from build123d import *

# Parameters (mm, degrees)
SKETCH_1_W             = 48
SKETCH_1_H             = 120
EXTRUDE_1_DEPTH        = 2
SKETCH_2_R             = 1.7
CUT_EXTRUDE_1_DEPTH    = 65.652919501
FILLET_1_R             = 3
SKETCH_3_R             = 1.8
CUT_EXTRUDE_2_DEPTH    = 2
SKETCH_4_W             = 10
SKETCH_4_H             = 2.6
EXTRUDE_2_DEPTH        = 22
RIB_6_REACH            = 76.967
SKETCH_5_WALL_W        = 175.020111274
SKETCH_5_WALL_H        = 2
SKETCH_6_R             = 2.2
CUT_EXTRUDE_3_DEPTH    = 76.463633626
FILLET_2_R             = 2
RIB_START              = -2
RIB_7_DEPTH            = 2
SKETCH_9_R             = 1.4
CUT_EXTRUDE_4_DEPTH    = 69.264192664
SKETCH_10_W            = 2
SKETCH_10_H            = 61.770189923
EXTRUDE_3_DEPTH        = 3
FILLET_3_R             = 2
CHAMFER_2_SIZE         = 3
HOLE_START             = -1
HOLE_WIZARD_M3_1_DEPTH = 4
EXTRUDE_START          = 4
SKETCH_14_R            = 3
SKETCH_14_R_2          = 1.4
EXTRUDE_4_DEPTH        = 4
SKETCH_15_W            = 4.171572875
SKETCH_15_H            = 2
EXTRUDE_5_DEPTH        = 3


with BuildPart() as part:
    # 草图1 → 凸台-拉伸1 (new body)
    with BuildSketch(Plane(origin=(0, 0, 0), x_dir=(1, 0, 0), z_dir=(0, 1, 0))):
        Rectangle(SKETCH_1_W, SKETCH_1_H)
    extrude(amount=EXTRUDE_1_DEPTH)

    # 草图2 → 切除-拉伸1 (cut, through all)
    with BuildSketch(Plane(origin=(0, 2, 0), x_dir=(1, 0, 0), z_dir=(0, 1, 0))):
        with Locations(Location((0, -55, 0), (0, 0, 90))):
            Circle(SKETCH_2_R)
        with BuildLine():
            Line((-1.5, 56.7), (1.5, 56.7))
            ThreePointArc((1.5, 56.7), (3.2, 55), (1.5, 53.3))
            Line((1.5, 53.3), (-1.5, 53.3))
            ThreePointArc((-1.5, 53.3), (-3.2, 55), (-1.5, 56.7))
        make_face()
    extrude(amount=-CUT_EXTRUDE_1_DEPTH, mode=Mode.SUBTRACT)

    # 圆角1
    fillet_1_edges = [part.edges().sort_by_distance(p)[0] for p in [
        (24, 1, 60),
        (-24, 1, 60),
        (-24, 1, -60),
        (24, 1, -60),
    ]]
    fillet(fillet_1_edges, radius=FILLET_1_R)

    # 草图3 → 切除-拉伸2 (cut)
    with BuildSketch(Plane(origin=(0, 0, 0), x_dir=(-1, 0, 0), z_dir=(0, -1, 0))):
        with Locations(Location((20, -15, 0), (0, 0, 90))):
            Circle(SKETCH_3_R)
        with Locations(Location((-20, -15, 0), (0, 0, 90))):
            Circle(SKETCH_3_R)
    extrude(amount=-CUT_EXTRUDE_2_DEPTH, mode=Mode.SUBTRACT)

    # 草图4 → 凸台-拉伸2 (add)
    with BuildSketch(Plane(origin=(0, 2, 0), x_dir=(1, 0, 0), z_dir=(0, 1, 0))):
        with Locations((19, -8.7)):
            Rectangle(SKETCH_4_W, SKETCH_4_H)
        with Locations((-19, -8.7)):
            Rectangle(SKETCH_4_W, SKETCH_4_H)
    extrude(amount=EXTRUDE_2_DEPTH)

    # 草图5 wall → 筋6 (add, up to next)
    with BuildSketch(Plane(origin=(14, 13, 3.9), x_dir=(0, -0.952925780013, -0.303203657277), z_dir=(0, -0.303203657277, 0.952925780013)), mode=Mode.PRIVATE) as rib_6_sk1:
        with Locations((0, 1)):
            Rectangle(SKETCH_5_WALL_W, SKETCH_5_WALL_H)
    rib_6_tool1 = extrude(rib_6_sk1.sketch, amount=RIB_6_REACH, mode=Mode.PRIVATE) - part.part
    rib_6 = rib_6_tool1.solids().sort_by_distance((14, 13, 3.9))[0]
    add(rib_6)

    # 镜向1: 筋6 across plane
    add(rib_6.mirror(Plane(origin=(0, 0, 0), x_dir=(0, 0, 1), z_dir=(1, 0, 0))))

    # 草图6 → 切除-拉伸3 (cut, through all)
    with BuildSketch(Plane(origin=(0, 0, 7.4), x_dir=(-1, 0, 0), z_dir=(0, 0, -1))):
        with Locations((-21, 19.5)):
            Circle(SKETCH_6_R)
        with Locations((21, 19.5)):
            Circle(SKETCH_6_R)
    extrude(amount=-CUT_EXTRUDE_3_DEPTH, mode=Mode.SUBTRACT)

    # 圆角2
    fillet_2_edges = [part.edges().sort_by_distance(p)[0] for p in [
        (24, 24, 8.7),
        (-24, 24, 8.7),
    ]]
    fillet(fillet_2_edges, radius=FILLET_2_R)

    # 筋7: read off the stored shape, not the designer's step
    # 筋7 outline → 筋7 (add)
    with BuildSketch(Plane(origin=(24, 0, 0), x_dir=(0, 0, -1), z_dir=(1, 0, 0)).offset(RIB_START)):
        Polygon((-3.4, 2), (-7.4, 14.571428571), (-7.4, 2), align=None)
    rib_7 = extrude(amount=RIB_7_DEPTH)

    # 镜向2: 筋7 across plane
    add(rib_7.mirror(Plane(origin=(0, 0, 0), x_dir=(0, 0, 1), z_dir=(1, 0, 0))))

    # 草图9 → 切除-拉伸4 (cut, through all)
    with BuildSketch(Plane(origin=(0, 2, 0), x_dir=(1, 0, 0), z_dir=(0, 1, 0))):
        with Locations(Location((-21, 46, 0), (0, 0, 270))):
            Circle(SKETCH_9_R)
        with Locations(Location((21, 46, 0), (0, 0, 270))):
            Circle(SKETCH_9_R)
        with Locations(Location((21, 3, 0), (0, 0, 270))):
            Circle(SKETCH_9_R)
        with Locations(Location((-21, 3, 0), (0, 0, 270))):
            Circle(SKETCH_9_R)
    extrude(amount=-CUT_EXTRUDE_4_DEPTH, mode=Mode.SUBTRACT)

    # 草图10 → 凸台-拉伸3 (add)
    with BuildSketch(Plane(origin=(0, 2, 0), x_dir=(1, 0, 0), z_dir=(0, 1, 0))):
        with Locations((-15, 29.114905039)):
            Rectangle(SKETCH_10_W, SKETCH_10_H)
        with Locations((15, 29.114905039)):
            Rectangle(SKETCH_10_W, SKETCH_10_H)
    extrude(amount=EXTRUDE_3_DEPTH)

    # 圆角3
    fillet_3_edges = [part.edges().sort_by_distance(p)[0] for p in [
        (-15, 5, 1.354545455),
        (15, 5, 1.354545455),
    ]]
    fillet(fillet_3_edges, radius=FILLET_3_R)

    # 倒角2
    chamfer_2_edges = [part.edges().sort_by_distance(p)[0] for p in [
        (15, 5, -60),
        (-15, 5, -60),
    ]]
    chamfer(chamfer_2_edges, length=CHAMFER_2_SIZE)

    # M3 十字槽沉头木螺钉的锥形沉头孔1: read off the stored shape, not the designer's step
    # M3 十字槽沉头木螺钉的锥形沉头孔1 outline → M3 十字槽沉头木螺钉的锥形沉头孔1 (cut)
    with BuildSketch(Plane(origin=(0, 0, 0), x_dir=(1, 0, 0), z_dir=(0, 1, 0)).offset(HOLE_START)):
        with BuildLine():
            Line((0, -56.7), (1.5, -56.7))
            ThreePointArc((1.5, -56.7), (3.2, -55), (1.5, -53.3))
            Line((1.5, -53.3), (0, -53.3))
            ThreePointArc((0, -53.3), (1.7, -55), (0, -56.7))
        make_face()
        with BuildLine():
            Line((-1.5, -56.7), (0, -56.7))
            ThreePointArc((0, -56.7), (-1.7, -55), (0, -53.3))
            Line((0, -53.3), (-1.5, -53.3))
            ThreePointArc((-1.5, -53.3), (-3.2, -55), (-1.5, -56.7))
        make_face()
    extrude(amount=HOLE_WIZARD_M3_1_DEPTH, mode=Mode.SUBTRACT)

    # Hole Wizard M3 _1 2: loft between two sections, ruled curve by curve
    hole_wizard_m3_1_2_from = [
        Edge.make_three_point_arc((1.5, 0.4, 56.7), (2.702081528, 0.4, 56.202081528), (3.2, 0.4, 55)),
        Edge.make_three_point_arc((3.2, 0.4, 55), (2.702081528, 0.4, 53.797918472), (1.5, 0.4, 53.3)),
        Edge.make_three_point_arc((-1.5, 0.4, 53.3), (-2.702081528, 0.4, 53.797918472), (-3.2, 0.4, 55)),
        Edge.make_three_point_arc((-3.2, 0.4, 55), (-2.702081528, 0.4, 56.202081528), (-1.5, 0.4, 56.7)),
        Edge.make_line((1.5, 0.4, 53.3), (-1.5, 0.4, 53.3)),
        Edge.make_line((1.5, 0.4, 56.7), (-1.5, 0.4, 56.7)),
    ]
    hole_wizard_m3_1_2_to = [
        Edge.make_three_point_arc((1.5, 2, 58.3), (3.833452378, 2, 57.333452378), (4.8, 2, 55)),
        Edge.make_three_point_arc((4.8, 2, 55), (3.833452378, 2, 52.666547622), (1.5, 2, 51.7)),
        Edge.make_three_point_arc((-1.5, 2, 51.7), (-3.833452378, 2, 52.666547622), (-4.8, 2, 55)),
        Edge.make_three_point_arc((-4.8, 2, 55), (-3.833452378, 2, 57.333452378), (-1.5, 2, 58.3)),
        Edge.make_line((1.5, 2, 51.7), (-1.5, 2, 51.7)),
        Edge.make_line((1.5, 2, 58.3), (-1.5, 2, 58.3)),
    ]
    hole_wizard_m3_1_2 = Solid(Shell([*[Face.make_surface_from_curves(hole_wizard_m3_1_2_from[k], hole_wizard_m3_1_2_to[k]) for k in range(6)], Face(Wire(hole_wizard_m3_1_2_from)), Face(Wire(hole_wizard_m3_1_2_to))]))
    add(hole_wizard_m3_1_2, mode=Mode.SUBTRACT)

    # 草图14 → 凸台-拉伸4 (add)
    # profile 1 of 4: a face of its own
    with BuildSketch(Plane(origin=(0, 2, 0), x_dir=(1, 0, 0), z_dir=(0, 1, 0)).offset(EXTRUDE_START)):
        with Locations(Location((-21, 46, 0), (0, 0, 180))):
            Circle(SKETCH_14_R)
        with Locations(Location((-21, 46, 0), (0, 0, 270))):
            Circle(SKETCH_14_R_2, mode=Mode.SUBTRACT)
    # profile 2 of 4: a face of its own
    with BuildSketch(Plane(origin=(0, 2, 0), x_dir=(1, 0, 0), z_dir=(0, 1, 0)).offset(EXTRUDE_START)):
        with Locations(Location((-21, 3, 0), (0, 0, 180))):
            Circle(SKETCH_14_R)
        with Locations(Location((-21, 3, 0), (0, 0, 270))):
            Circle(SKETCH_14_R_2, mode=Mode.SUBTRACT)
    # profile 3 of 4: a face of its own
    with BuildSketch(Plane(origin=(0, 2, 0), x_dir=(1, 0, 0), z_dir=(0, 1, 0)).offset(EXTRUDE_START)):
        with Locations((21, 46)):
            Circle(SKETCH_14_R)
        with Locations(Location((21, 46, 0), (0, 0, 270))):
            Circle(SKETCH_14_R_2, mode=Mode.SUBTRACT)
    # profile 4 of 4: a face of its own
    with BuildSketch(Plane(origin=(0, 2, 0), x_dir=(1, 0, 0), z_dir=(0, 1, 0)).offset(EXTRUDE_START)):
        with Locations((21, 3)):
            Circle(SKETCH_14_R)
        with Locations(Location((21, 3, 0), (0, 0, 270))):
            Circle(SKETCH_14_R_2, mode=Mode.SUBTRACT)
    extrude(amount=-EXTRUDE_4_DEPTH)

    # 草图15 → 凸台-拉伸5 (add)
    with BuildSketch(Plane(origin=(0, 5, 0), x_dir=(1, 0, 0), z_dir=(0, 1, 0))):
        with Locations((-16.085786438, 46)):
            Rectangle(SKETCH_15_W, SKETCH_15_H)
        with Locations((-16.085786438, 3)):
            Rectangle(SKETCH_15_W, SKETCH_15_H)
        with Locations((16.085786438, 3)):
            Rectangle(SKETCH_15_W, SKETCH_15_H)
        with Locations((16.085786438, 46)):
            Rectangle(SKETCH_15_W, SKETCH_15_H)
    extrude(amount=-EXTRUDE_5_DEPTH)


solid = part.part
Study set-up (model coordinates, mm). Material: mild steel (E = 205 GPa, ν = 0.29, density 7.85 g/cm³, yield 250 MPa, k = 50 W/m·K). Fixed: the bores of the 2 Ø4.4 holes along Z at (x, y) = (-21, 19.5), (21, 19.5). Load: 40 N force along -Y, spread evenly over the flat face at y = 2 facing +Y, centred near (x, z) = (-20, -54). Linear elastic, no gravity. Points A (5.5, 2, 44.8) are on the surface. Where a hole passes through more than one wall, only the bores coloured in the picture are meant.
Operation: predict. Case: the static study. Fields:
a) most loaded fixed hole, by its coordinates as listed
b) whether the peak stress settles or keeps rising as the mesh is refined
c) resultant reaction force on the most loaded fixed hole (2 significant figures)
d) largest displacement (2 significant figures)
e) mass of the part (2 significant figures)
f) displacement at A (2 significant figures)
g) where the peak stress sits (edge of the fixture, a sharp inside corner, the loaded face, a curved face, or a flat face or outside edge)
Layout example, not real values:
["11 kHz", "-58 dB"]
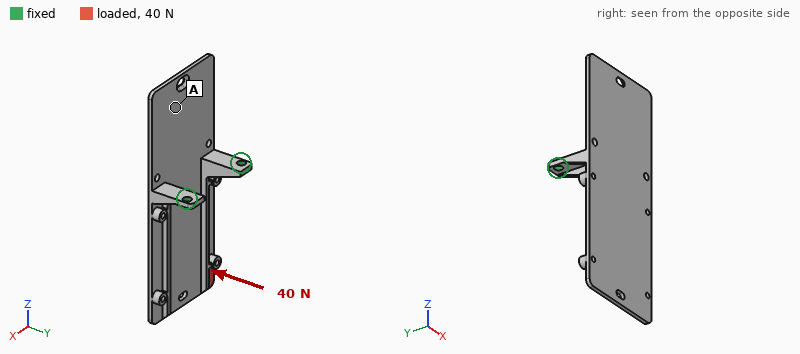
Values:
["(-21, 19.5)", "keeps rising", "46 N", "0.32 mm", "110 g", "0.069 mm", "edge of the fixture"]
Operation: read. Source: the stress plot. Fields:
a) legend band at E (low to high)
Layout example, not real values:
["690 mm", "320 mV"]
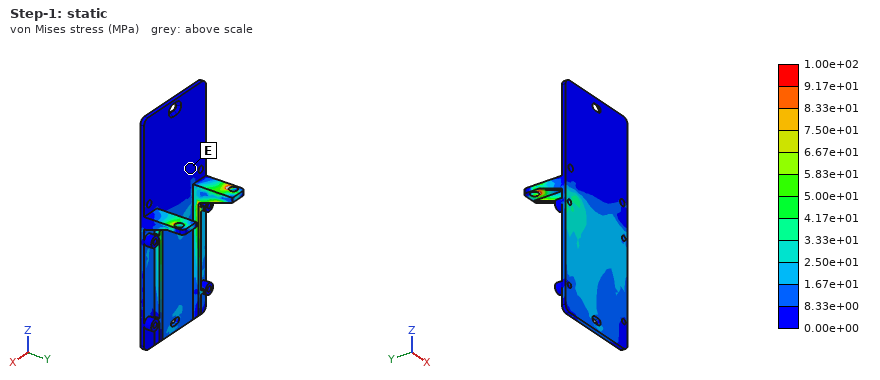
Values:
["0.00e+00 to 8.33e+00 MPa"]
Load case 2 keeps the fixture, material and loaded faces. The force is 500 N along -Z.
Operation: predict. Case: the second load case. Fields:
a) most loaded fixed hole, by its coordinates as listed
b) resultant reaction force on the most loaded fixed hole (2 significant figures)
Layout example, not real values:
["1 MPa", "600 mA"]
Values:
["(-21, 19.5)", "480 N"]
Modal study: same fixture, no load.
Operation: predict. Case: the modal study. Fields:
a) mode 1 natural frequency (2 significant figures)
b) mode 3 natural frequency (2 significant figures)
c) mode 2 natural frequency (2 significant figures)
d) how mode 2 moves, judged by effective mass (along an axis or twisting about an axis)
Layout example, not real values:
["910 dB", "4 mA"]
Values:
["410 Hz", "870 Hz", "630 Hz", "along Y"]
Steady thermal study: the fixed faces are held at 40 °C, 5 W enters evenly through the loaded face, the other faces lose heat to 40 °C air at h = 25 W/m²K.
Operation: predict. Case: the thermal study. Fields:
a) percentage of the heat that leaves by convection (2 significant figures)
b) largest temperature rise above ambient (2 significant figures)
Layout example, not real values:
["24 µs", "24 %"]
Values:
["81 %", "61 K"]
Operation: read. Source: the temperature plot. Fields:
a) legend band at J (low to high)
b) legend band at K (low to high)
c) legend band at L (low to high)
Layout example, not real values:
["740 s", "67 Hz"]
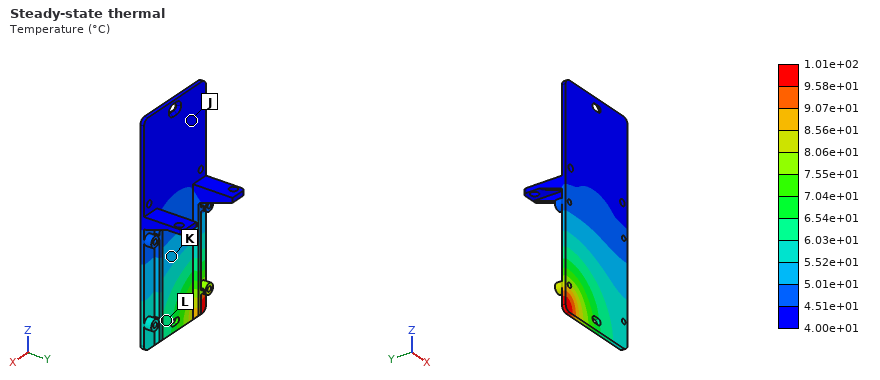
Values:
["4.00e+01 to 4.51e+01 °C", "5.01e+01 to 5.52e+01 °C", "6.03e+01 to 6.54e+01 °C"]
